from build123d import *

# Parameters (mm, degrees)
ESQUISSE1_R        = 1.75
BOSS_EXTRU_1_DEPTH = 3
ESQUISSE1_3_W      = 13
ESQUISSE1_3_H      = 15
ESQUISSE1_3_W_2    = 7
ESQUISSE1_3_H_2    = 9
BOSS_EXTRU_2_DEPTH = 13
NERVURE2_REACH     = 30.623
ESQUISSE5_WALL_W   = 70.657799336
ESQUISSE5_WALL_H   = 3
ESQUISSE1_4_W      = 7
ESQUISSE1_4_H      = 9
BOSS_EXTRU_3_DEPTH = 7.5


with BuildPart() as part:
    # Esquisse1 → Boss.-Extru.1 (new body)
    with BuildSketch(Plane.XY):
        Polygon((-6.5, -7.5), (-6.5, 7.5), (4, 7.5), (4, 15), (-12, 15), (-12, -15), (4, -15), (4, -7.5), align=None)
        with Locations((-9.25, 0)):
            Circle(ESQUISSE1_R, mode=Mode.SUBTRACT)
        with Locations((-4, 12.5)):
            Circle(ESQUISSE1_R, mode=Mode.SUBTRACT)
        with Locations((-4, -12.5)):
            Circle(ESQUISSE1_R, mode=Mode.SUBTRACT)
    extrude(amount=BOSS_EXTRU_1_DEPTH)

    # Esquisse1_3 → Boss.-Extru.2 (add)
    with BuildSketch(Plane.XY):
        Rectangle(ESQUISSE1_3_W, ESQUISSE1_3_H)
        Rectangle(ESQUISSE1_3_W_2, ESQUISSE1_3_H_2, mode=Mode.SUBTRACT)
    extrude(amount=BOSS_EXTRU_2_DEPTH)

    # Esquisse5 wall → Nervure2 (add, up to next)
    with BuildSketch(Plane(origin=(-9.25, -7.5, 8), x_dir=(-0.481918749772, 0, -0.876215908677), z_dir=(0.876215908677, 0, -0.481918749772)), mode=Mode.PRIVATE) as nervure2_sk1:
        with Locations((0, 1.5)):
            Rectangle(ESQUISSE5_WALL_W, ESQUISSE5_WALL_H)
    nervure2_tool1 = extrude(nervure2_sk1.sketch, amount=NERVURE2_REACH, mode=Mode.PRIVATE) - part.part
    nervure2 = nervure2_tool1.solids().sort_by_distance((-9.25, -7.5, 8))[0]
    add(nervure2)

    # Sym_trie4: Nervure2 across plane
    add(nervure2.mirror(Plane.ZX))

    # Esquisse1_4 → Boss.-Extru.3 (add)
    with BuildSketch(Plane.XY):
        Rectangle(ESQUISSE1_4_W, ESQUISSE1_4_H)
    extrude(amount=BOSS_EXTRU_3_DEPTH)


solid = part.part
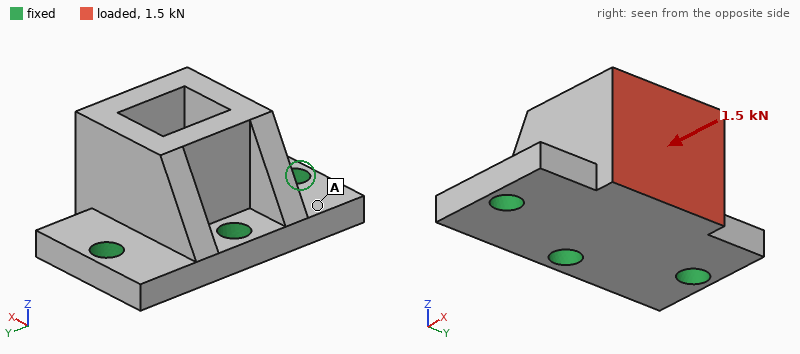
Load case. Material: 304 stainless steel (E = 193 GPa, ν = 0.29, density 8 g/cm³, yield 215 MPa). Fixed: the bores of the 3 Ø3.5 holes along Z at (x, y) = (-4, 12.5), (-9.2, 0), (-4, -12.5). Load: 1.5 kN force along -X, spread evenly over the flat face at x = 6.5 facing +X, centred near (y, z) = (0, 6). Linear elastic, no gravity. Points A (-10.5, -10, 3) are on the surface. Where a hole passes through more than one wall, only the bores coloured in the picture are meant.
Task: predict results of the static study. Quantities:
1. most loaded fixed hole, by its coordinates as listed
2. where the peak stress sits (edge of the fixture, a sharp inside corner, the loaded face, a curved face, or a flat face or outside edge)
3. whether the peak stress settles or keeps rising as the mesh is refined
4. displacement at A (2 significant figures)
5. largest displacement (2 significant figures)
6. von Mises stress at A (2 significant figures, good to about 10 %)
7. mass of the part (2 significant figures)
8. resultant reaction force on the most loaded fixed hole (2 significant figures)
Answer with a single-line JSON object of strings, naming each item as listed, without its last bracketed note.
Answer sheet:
{"most loaded fixed hole, by its coordinates as listed": "(-9.2, 0)", "where the peak stress sits": "edge of the fixture", "whether the peak stress settles or keeps rising as the mesh is refined": "keeps rising", "displacement at A": "2.5 µm", "largest displacement": "17 µm", "von Mises stress at A": "20 MPa", "mass of the part": "26 g", "resultant reaction force on the most loaded fixed hole": "1.1 kN"}
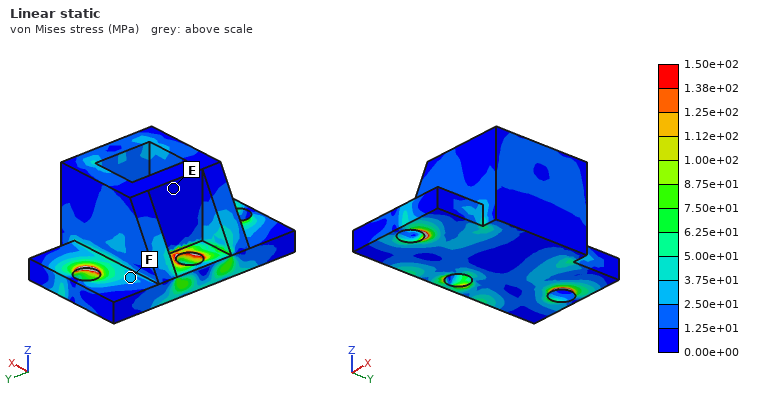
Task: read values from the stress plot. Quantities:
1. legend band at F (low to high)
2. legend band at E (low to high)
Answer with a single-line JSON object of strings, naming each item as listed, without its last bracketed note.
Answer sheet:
{"legend band at F": "2.50e+01 to 3.75e+01 MPa", "legend band at E": "0.00e+00 to 1.25e+01 MPa"}
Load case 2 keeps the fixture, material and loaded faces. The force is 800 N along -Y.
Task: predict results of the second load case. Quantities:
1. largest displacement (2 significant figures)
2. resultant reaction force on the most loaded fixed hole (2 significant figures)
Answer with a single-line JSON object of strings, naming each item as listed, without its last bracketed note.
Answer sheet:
{"largest displacement": "4.0 µm", "resultant reaction force on the most loaded fixed hole": "520 N"}
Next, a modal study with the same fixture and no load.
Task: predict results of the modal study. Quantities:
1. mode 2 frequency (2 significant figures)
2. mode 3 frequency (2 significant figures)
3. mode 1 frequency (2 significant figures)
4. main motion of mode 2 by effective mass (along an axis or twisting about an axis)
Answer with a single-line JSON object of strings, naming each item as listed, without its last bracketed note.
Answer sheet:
{"mode 2 frequency": "25 kHz", "mode 3 frequency": "38 kHz", "mode 1 frequency": "12 kHz", "main motion of mode 2 by effective mass": "along Y"}
